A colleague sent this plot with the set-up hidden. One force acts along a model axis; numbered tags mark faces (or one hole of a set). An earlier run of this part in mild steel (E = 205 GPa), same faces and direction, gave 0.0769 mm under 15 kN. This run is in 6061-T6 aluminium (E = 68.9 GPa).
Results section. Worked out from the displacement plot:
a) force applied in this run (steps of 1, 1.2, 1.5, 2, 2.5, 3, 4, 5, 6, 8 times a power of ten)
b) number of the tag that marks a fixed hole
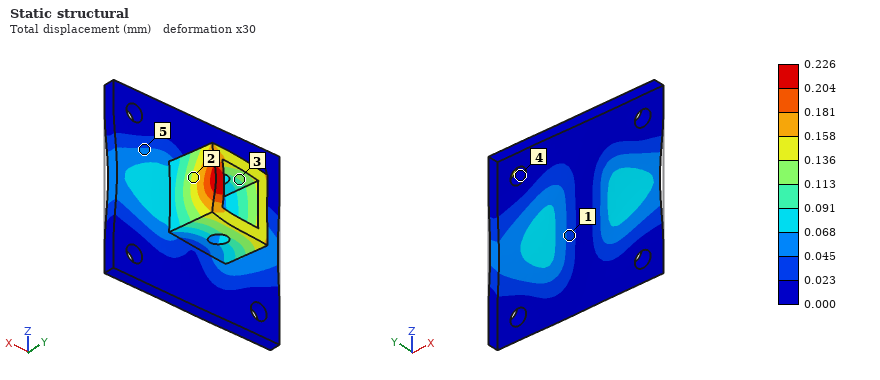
15 kN
4
